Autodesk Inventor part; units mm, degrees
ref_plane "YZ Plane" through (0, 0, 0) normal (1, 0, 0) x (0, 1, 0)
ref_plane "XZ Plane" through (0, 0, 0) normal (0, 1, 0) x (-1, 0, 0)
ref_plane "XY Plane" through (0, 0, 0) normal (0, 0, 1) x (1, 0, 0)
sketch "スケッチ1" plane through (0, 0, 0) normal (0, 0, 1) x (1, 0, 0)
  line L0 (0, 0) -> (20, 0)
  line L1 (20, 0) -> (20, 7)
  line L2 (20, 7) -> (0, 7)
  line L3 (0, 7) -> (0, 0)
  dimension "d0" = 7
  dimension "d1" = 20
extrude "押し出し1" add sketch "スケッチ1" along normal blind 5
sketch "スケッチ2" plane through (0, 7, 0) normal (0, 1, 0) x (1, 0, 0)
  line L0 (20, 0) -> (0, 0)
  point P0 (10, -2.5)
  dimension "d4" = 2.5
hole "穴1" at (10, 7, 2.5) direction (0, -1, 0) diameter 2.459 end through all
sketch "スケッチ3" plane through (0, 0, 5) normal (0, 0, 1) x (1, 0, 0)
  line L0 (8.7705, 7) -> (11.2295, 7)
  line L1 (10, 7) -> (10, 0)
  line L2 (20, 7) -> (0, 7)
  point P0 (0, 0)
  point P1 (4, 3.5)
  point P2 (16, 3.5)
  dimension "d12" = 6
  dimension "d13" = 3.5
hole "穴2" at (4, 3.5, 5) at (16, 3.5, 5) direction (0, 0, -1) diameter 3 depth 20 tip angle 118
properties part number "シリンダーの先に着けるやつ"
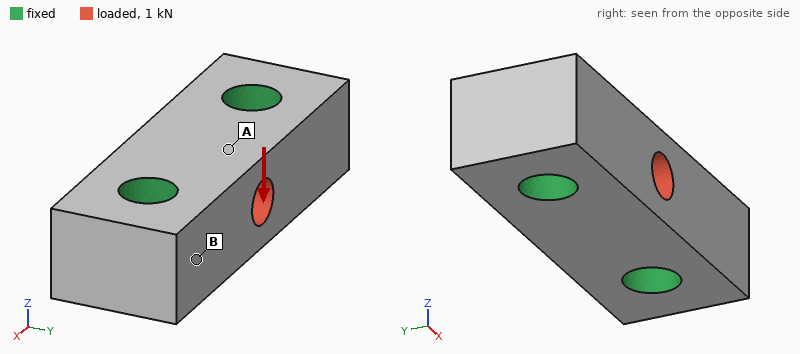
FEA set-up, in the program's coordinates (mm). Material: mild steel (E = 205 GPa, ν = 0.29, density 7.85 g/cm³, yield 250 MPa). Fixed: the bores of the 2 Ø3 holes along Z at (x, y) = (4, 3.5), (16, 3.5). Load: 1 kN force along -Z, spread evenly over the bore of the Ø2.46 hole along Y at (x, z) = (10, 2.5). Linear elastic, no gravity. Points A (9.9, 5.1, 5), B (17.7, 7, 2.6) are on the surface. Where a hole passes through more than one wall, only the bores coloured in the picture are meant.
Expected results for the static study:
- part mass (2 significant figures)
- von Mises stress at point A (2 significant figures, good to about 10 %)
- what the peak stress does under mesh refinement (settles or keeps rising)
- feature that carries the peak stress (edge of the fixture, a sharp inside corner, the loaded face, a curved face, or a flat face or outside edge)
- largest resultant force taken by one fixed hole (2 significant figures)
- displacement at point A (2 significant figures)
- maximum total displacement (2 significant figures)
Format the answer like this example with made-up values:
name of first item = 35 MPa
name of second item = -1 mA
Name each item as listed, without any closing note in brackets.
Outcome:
part mass = 4.7 g
von Mises stress at point A = 50 MPa
what the peak stress does under mesh refinement = keeps rising
feature that carries the peak stress = edge of the fixture
largest resultant force taken by one fixed hole = 500 N
displacement at point A = 1.3 µm
maximum total displacement = 1.5 µm
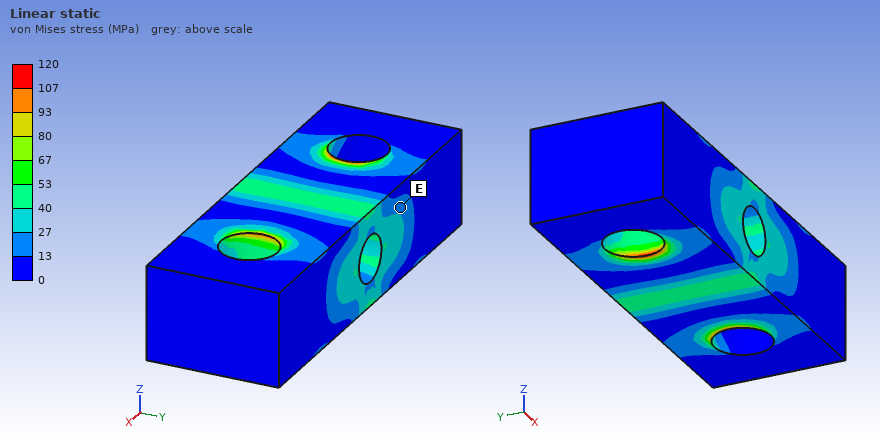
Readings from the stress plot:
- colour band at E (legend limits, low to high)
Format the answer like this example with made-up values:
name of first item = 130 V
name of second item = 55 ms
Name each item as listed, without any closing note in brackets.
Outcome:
colour band at E = 13 to 27 MPa
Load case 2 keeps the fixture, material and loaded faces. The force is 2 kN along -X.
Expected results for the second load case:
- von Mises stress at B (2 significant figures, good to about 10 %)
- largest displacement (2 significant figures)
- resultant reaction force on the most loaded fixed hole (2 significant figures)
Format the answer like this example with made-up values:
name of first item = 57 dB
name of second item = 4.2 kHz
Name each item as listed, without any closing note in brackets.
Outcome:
von Mises stress at B = 5.5 MPa
largest displacement = 0.84 µm
resultant reaction force on the most loaded fixed hole = 1.0 kN
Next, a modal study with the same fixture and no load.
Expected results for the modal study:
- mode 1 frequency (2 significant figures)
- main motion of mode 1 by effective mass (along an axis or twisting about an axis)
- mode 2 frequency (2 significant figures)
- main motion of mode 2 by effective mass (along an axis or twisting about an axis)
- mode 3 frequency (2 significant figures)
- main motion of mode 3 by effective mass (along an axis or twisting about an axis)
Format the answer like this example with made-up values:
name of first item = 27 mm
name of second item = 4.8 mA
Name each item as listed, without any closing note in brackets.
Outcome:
mode 1 frequency = 120 kHz
main motion of mode 1 by effective mass = along Y
mode 2 frequency = 130 kHz
main motion of mode 2 by effective mass = along Z
mode 3 frequency = 140 kHz
main motion of mode 3 by effective mass = twisting about X
